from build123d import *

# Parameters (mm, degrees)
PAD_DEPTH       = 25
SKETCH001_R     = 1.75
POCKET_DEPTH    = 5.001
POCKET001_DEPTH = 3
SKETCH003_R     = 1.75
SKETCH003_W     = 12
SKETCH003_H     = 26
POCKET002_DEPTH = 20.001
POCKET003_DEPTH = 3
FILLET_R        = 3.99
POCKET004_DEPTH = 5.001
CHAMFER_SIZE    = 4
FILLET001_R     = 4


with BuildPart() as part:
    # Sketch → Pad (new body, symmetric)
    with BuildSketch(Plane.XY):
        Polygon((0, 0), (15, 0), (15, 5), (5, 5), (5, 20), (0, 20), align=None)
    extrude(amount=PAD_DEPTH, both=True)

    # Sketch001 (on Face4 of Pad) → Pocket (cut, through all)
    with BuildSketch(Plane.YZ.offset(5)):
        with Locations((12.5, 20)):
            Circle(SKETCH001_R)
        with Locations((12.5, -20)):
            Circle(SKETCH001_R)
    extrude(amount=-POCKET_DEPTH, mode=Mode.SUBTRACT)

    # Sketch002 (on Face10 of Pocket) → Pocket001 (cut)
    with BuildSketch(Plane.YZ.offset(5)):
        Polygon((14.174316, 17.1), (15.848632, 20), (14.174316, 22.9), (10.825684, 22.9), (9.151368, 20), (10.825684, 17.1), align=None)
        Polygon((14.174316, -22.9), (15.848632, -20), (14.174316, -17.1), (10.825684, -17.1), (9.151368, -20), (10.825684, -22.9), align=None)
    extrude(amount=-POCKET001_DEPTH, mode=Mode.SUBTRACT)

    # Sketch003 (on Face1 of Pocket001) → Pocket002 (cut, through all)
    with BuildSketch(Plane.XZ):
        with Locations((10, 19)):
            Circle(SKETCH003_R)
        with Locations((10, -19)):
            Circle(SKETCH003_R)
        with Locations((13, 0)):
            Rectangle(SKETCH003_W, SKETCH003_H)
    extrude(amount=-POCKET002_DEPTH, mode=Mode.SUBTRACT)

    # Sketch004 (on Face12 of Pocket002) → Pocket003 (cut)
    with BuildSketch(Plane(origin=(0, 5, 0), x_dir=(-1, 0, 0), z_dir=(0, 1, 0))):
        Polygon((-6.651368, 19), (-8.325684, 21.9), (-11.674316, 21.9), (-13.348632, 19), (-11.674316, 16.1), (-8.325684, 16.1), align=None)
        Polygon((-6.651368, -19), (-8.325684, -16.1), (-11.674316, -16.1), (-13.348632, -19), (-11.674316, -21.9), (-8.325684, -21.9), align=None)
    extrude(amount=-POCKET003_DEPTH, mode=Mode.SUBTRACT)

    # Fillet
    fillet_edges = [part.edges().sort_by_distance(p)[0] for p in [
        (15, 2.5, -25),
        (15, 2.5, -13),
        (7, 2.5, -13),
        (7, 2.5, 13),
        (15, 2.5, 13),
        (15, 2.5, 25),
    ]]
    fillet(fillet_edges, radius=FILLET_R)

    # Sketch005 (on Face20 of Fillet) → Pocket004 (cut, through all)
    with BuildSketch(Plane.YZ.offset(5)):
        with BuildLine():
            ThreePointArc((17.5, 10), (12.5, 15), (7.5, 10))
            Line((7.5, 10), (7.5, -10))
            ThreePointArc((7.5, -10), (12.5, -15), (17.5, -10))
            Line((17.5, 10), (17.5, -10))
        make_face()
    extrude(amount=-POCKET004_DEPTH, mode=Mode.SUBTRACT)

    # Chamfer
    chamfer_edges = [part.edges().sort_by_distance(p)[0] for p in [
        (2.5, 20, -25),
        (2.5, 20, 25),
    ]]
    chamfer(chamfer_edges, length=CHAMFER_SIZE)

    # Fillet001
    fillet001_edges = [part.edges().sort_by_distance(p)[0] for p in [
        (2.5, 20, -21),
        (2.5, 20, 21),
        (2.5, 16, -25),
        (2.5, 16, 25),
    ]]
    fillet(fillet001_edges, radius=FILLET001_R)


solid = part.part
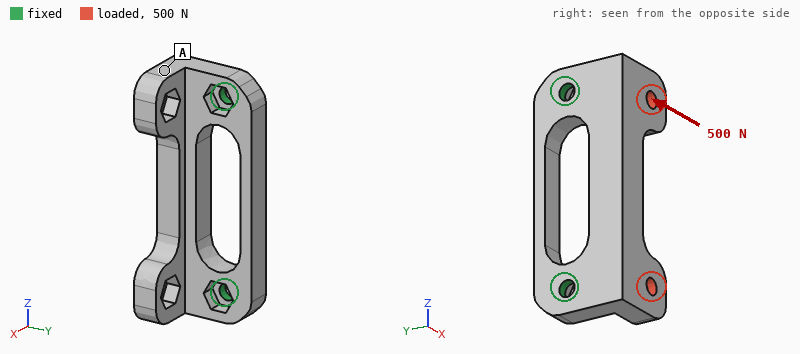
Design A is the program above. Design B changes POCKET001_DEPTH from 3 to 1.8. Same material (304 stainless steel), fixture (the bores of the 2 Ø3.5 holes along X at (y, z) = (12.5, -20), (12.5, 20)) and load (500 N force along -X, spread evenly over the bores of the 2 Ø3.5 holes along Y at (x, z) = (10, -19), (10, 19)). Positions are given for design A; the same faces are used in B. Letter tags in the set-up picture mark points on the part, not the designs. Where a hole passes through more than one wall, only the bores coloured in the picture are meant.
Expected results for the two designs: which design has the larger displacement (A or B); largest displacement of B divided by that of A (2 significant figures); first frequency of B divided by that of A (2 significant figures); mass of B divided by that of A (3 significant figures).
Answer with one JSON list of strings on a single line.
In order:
["A", "0.60", "1.3", "1.01"]
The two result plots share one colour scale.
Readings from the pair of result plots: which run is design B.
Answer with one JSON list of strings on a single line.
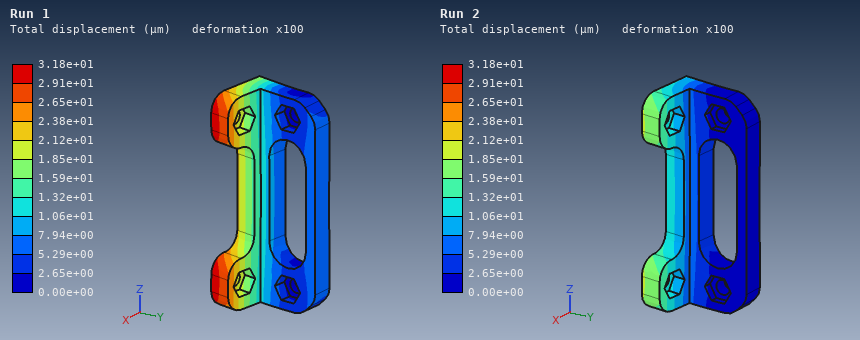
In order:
["Run 2"]
